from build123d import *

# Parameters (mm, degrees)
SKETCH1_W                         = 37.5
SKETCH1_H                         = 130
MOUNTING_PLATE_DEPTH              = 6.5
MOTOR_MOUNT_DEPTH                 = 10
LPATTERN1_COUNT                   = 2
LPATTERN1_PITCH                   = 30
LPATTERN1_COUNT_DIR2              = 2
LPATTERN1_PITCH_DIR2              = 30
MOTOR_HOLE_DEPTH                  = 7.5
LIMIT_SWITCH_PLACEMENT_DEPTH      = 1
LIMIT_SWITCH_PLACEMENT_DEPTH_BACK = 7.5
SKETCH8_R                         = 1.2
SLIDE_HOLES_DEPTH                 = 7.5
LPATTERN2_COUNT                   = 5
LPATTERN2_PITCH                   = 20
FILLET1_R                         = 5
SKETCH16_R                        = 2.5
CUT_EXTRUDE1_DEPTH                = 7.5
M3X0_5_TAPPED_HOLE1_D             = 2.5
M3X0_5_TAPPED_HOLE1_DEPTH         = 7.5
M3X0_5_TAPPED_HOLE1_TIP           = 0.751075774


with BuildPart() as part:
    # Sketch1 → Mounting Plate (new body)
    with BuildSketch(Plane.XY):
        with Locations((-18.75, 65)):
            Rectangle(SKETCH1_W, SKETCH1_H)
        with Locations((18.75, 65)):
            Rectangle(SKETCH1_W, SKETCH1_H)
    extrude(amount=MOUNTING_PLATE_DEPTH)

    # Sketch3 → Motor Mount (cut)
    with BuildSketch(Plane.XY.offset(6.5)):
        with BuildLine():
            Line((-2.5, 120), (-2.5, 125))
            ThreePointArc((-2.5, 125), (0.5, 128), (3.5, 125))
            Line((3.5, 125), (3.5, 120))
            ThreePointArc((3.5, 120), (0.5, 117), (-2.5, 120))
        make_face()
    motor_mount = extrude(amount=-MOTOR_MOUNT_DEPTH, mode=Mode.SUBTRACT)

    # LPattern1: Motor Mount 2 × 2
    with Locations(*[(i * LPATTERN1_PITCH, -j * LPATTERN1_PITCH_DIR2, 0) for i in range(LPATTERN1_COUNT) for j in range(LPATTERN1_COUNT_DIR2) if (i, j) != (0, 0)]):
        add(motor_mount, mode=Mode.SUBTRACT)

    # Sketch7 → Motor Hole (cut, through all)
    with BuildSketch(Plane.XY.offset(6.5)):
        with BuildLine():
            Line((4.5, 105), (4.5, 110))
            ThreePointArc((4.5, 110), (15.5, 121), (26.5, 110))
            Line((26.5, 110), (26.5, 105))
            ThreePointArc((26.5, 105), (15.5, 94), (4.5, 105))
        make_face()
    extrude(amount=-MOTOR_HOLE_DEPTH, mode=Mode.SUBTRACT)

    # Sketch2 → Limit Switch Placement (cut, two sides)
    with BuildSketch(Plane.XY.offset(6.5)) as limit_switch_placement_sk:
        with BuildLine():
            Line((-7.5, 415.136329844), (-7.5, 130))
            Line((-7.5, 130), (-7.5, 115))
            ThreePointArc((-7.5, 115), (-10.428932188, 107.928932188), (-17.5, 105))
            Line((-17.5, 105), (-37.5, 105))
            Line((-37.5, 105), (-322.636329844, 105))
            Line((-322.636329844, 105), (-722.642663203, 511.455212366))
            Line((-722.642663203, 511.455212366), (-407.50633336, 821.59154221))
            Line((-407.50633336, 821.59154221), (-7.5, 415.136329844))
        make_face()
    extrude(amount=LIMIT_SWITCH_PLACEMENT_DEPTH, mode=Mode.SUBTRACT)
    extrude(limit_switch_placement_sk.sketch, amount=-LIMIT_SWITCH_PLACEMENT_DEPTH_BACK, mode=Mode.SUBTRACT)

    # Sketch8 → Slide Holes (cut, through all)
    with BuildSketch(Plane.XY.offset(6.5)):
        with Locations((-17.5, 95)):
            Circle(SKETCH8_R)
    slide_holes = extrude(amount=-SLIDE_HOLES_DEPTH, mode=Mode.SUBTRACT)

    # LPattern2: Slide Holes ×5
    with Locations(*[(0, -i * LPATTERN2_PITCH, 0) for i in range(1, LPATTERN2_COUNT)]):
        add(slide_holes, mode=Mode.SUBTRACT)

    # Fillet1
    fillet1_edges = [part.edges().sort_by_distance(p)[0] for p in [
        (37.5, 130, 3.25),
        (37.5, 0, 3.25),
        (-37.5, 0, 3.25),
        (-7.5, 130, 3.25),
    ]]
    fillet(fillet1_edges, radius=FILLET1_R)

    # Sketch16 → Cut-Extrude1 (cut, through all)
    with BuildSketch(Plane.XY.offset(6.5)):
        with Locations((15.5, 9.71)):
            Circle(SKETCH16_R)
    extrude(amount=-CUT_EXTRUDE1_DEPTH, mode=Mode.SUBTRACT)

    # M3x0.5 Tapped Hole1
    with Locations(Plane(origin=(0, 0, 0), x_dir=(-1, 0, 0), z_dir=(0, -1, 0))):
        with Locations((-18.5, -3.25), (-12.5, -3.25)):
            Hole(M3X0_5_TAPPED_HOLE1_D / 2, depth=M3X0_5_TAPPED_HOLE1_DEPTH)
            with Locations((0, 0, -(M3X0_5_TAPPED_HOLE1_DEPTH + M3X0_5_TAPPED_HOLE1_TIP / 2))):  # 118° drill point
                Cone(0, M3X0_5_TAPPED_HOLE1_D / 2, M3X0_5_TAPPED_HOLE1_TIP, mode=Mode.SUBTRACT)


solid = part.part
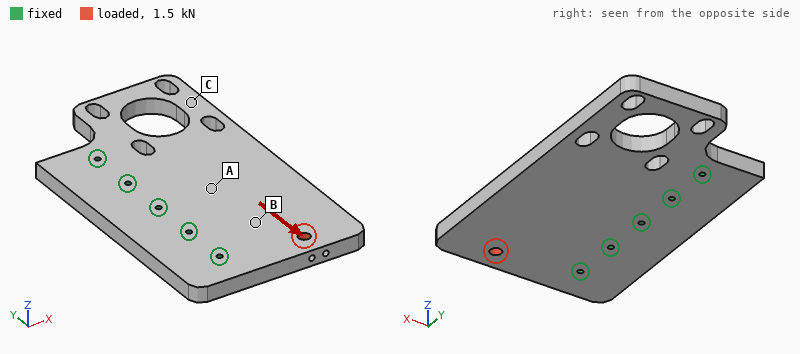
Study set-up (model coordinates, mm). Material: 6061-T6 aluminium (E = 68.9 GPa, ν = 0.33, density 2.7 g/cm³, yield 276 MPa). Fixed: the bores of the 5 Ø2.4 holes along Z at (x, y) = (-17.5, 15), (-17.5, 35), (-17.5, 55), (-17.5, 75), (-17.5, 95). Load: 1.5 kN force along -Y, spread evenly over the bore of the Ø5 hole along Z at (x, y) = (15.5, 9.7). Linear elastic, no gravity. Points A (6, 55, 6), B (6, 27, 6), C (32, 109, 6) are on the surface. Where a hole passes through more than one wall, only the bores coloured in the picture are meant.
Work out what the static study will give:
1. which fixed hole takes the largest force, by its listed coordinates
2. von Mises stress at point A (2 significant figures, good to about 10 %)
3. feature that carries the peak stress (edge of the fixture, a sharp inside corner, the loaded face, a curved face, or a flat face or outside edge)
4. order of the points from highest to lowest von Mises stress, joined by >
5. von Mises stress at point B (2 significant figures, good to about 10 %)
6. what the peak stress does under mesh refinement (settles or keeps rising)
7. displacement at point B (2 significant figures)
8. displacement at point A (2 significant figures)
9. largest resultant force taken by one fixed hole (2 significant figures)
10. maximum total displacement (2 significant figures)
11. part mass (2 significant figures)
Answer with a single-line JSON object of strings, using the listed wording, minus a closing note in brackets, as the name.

{"which fixed hole takes the largest force, by its listed coordinates": "(-17.5, 15)", "von Mises stress at point A": "4.5 MPa", "feature that carries the peak stress": "edge of the fixture", "order of the points from highest to lowest von Mises stress, joined by >": "B > A > C", "von Mises stress at point B": "7.7 MPa", "what the peak stress does under mesh refinement": "keeps rising", "displacement at point B": "4.1 µm", "displacement at point A": "2.7 µm", "largest resultant force taken by one fixed hole": "790 N", "maximum total displacement": "9.4 µm", "part mass": "140 g"}
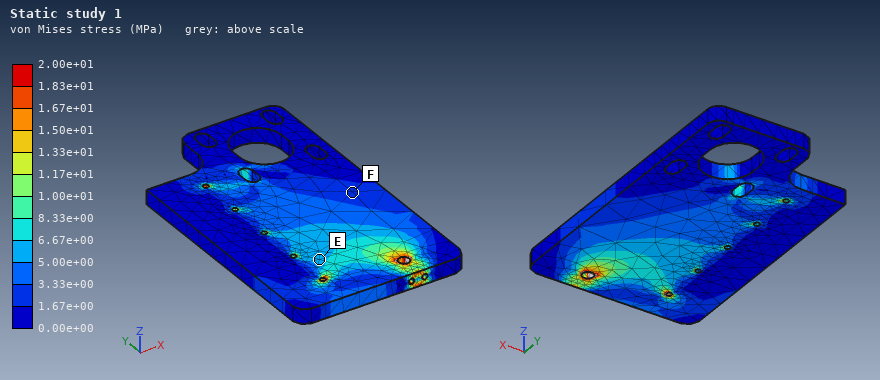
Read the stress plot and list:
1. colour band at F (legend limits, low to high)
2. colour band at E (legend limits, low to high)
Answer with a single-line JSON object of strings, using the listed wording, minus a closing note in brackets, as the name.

{"colour band at F": "1.67e+00 to 3.33e+00 MPa", "colour band at E": "5.00e+00 to 6.67e+00 MPa"}
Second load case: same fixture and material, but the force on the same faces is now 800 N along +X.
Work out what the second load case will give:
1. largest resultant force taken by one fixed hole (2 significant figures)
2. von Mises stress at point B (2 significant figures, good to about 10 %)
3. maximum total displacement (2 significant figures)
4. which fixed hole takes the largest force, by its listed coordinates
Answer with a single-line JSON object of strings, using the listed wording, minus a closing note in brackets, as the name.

{"largest resultant force taken by one fixed hole": "660 N", "von Mises stress at point B": "2.1 MPa", "maximum total displacement": "4.4 µm", "which fixed hole takes the largest force, by its listed coordinates": "(-17.5, 15)"}
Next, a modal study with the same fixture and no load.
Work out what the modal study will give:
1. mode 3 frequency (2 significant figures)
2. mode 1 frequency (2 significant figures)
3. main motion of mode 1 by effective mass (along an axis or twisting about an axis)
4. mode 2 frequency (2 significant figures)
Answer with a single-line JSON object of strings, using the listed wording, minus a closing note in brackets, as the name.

{"mode 3 frequency": "3300 Hz", "mode 1 frequency": "1500 Hz", "main motion of mode 1 by effective mass": "along Z", "mode 2 frequency": "2000 Hz"}
